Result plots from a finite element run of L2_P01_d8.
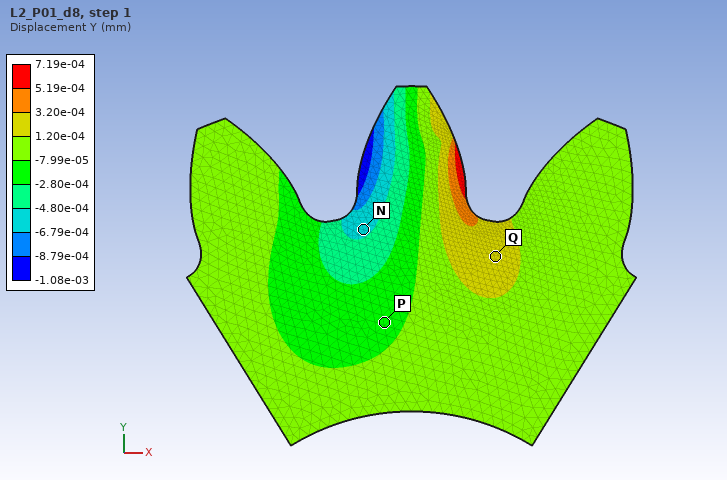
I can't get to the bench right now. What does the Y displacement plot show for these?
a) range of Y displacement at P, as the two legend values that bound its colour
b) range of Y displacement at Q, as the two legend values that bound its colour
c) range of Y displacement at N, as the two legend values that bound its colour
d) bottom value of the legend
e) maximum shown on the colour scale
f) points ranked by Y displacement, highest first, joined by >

-2.80e-04 to -7.99e-05 mm
1.20e-04 to 3.20e-04 mm
-6.79e-04 to -4.80e-04 mm
-1.08e-03 mm
7.19e-04 mm
Q > P > N
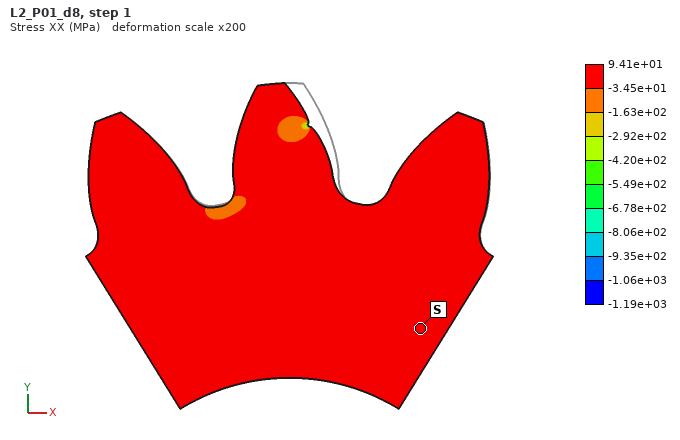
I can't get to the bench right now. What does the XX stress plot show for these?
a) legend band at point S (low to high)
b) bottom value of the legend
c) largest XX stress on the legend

-3.45e+01 to 9.41e+01 MPa
-1.19e+03 MPa
9.41e+01 MPa
